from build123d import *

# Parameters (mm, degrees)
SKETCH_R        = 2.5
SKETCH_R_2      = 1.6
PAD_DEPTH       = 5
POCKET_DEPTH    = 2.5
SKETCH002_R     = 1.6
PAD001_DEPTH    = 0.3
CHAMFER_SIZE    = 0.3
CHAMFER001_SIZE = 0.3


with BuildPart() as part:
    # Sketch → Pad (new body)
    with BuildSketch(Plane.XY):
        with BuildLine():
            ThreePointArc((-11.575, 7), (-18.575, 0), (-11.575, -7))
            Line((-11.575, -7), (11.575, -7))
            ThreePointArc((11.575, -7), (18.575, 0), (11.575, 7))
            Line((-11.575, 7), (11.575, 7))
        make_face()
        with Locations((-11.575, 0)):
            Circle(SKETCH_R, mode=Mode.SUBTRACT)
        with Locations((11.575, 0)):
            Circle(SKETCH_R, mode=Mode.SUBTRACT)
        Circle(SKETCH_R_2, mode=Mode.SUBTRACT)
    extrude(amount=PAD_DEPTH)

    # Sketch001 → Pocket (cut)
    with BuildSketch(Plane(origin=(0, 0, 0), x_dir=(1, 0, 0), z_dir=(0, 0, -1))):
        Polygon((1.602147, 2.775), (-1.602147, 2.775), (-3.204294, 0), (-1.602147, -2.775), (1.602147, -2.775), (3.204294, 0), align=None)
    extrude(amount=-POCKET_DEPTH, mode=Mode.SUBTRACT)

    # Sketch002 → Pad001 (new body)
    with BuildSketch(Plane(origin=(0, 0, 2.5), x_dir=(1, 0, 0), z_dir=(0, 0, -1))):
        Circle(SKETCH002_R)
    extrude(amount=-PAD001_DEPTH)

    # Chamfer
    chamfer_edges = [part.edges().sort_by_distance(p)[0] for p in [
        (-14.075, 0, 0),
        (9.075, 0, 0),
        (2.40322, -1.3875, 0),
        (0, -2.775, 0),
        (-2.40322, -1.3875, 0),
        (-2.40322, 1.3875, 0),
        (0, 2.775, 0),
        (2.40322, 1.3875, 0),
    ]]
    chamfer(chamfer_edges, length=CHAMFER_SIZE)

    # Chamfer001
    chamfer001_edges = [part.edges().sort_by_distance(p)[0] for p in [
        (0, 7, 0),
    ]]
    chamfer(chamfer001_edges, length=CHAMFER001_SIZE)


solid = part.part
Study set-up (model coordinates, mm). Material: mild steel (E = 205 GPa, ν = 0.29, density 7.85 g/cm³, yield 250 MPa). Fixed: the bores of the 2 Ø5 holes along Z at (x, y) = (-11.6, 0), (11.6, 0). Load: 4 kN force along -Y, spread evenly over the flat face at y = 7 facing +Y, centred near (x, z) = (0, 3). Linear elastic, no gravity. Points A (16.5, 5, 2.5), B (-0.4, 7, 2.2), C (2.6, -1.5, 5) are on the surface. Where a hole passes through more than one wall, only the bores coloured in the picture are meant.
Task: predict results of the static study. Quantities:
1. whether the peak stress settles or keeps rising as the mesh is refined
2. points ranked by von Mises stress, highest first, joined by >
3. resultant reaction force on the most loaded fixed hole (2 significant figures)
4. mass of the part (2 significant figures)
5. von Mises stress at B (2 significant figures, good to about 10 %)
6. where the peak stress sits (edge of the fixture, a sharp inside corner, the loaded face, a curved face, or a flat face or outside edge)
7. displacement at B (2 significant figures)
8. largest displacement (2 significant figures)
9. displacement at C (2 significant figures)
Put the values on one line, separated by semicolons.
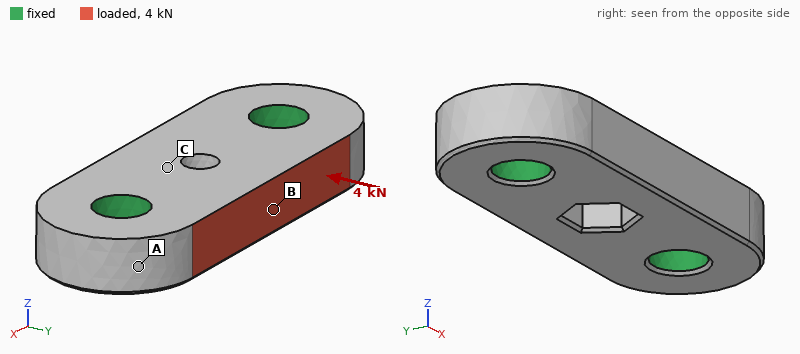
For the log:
keeps rising; B > C > A; 2.0 kN; 17 g; 52 MPa; edge of the fixture; 3.7 µm; 3.8 µm; 2.4 µm
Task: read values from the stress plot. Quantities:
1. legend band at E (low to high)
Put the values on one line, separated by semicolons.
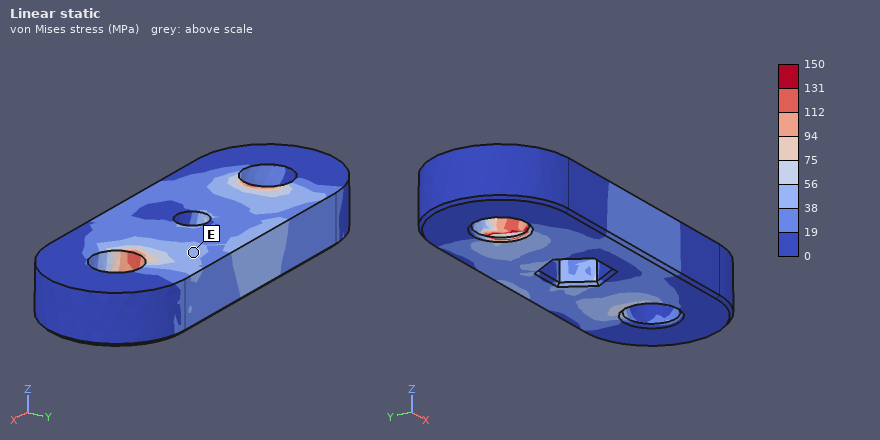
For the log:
38 to 56 MPa
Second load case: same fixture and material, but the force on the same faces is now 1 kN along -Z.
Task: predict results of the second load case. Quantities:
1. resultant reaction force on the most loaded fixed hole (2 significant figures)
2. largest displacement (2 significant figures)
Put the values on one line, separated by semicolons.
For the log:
500 N; 5.9 µm
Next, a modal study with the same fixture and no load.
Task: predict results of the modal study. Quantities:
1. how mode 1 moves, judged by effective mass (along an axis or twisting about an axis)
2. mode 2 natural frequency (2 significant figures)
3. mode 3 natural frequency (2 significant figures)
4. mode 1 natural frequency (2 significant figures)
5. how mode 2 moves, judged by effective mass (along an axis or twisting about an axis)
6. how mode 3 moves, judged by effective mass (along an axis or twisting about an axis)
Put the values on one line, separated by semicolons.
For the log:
along Z; 48 kHz; 62 kHz; 44 kHz; twisting about X; along Y
